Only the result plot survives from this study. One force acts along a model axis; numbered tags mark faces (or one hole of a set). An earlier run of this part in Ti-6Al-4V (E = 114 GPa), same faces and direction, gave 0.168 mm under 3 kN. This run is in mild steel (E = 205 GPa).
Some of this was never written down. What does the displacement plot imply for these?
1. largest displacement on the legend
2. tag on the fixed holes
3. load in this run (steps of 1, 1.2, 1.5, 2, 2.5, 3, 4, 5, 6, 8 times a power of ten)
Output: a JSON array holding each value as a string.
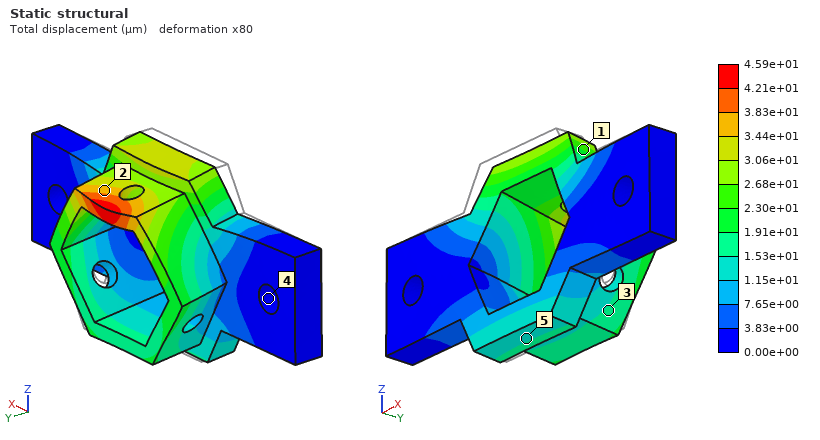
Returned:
["4.59e+01 µm", "4", "1.5 kN"]
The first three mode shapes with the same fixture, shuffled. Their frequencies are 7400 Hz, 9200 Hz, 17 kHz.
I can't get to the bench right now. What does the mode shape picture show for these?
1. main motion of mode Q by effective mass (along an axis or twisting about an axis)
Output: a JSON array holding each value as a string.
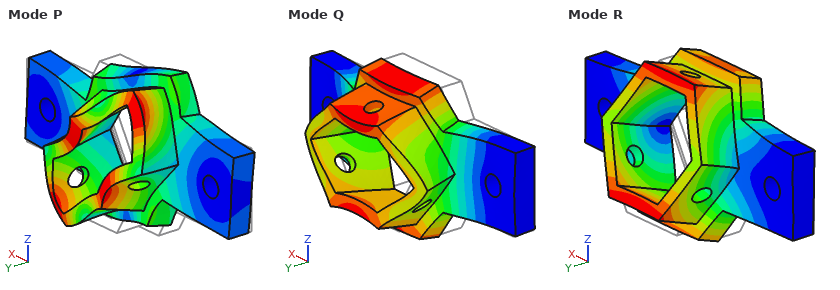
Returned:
["along Y"]
